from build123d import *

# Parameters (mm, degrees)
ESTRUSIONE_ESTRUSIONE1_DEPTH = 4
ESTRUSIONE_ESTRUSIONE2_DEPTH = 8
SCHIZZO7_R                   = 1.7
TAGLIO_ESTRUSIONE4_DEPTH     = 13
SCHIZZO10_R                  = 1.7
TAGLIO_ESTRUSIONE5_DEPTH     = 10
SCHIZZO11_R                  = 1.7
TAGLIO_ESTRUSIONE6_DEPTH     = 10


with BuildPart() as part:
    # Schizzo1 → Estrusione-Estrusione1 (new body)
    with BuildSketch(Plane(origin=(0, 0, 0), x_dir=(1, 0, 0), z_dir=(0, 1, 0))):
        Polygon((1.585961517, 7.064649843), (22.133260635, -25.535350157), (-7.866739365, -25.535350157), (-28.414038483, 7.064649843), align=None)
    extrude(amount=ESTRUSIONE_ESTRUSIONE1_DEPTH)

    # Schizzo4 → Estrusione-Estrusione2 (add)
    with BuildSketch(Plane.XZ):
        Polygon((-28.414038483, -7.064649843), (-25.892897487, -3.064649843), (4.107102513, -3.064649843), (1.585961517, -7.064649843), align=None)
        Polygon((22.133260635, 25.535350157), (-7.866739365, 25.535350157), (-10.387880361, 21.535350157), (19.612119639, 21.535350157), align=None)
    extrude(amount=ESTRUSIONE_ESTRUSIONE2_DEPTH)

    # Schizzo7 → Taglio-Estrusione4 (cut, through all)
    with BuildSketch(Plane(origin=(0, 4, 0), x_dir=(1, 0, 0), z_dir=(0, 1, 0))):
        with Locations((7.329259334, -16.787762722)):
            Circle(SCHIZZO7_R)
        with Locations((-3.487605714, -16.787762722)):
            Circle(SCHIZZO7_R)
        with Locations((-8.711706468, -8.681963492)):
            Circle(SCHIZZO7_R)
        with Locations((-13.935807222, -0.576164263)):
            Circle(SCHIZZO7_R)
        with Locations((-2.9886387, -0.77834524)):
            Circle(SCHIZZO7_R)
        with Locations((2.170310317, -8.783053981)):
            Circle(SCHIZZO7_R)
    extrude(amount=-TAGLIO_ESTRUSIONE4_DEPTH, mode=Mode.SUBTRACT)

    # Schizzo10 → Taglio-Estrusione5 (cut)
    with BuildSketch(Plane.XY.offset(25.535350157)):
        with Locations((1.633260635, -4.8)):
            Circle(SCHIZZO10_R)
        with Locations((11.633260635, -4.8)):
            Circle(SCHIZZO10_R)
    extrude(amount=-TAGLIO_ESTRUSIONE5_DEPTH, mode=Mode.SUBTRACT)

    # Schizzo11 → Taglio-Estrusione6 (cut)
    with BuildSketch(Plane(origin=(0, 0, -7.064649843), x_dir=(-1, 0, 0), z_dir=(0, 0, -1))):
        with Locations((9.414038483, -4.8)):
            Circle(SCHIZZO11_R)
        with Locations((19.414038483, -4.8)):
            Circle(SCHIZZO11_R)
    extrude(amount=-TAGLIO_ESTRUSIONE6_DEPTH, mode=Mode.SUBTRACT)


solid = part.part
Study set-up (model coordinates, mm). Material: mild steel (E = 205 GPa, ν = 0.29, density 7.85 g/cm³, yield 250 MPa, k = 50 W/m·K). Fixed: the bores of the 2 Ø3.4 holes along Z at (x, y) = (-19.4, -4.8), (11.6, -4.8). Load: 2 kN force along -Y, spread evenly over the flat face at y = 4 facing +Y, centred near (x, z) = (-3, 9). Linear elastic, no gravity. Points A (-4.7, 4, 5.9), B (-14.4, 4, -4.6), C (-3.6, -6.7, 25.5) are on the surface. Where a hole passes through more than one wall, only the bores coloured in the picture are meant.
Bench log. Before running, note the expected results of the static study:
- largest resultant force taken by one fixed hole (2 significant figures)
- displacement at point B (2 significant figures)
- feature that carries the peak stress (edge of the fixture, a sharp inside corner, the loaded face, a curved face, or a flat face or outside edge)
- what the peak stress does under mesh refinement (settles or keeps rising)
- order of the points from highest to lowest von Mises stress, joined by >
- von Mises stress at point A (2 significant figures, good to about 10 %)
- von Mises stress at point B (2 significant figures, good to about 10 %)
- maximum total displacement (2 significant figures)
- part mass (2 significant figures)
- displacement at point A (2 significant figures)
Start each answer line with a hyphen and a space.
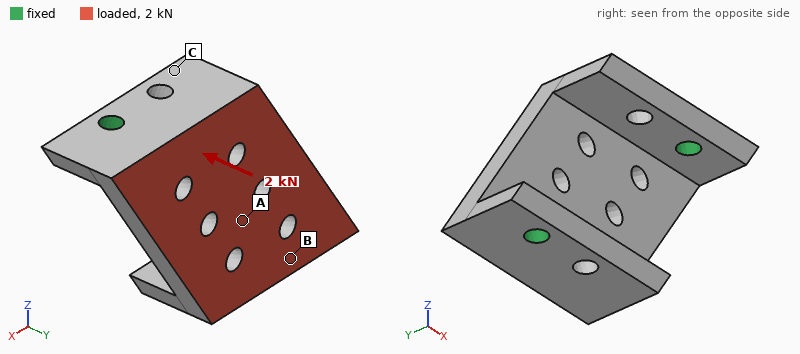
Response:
- 1.4 kN
- 4.1 µm
- edge of the fixture
- keeps rising
- A > B > C
- 54 MPa
- 26 MPa
- 17 µm
- 43 g
- 14 µm
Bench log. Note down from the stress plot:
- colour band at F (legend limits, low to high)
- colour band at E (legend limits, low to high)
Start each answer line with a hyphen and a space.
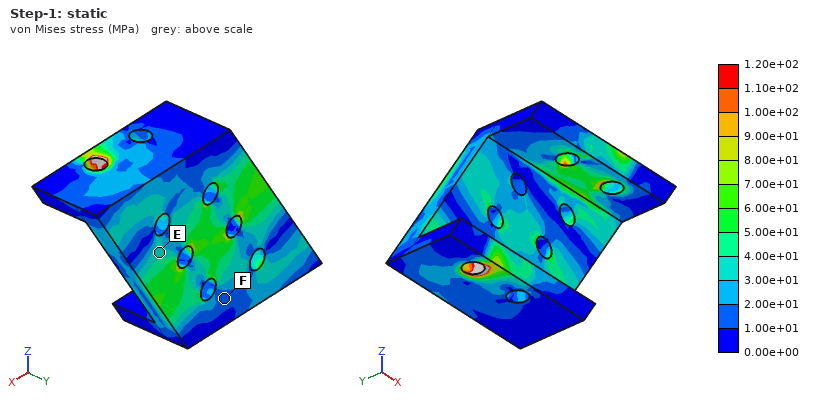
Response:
- 1.00e+01 to 2.00e+01 MPa
- 3.00e+01 to 4.00e+01 MPa
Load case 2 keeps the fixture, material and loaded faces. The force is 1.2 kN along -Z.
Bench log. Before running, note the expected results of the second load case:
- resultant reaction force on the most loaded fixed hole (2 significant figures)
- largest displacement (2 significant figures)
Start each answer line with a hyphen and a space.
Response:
- 630 N
- 10 µm
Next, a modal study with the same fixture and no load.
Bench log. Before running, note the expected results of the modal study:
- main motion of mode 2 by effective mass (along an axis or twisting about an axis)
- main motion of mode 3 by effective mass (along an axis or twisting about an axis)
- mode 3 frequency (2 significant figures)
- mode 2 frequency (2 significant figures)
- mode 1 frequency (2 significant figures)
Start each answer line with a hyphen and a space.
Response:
- along Y
- along Z
- 14 kHz
- 11 kHz
- 8800 Hz
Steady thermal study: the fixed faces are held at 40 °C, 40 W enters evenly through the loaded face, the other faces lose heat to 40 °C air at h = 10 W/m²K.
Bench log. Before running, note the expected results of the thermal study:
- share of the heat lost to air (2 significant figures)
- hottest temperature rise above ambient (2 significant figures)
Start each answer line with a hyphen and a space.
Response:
- 3.6 %
- 81 K
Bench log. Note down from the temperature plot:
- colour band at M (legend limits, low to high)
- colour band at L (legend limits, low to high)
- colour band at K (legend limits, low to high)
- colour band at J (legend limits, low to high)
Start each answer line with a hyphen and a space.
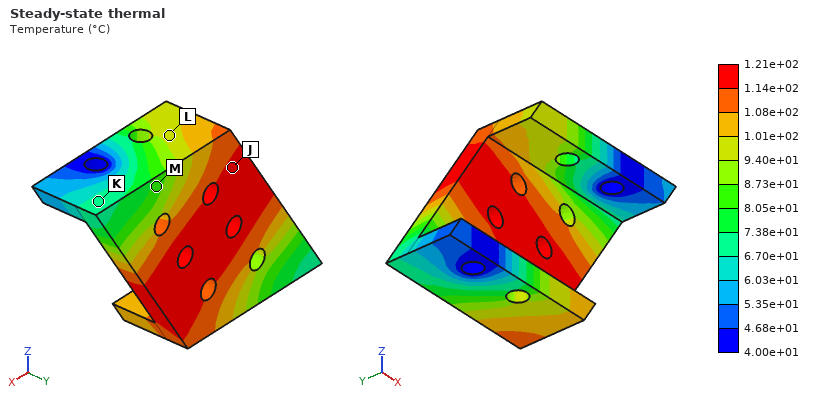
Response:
- 8.05e+01 to 8.73e+01 °C
- 9.40e+01 to 1.01e+02 °C
- 6.70e+01 to 7.38e+01 °C
- 1.14e+02 to 1.21e+02 °C
